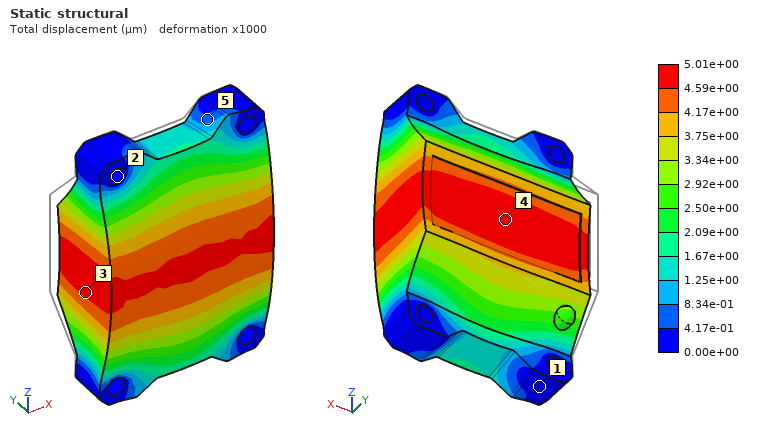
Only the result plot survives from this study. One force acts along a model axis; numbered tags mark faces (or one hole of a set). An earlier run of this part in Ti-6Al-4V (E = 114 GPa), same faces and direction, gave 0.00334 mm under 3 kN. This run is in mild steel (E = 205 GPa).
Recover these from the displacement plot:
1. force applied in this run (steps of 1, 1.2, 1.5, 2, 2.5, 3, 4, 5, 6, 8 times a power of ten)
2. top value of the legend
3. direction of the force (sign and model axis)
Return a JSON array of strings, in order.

["8 kN", "5.01e+00 µm", "-Y"]
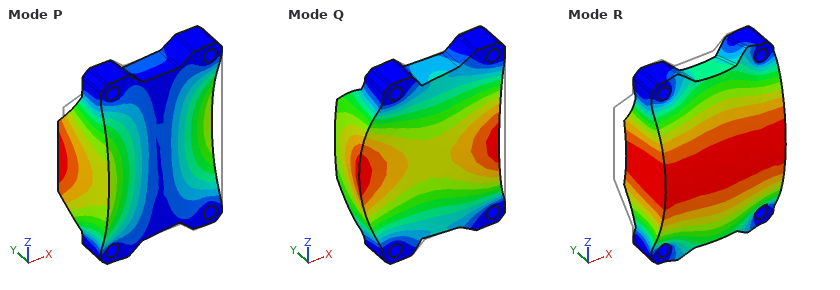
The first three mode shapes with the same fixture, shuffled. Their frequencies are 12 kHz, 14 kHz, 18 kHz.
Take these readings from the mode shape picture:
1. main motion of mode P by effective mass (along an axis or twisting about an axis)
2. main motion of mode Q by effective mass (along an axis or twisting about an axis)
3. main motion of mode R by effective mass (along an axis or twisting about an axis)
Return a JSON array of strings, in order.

["along X", "along X", "along Y"]
